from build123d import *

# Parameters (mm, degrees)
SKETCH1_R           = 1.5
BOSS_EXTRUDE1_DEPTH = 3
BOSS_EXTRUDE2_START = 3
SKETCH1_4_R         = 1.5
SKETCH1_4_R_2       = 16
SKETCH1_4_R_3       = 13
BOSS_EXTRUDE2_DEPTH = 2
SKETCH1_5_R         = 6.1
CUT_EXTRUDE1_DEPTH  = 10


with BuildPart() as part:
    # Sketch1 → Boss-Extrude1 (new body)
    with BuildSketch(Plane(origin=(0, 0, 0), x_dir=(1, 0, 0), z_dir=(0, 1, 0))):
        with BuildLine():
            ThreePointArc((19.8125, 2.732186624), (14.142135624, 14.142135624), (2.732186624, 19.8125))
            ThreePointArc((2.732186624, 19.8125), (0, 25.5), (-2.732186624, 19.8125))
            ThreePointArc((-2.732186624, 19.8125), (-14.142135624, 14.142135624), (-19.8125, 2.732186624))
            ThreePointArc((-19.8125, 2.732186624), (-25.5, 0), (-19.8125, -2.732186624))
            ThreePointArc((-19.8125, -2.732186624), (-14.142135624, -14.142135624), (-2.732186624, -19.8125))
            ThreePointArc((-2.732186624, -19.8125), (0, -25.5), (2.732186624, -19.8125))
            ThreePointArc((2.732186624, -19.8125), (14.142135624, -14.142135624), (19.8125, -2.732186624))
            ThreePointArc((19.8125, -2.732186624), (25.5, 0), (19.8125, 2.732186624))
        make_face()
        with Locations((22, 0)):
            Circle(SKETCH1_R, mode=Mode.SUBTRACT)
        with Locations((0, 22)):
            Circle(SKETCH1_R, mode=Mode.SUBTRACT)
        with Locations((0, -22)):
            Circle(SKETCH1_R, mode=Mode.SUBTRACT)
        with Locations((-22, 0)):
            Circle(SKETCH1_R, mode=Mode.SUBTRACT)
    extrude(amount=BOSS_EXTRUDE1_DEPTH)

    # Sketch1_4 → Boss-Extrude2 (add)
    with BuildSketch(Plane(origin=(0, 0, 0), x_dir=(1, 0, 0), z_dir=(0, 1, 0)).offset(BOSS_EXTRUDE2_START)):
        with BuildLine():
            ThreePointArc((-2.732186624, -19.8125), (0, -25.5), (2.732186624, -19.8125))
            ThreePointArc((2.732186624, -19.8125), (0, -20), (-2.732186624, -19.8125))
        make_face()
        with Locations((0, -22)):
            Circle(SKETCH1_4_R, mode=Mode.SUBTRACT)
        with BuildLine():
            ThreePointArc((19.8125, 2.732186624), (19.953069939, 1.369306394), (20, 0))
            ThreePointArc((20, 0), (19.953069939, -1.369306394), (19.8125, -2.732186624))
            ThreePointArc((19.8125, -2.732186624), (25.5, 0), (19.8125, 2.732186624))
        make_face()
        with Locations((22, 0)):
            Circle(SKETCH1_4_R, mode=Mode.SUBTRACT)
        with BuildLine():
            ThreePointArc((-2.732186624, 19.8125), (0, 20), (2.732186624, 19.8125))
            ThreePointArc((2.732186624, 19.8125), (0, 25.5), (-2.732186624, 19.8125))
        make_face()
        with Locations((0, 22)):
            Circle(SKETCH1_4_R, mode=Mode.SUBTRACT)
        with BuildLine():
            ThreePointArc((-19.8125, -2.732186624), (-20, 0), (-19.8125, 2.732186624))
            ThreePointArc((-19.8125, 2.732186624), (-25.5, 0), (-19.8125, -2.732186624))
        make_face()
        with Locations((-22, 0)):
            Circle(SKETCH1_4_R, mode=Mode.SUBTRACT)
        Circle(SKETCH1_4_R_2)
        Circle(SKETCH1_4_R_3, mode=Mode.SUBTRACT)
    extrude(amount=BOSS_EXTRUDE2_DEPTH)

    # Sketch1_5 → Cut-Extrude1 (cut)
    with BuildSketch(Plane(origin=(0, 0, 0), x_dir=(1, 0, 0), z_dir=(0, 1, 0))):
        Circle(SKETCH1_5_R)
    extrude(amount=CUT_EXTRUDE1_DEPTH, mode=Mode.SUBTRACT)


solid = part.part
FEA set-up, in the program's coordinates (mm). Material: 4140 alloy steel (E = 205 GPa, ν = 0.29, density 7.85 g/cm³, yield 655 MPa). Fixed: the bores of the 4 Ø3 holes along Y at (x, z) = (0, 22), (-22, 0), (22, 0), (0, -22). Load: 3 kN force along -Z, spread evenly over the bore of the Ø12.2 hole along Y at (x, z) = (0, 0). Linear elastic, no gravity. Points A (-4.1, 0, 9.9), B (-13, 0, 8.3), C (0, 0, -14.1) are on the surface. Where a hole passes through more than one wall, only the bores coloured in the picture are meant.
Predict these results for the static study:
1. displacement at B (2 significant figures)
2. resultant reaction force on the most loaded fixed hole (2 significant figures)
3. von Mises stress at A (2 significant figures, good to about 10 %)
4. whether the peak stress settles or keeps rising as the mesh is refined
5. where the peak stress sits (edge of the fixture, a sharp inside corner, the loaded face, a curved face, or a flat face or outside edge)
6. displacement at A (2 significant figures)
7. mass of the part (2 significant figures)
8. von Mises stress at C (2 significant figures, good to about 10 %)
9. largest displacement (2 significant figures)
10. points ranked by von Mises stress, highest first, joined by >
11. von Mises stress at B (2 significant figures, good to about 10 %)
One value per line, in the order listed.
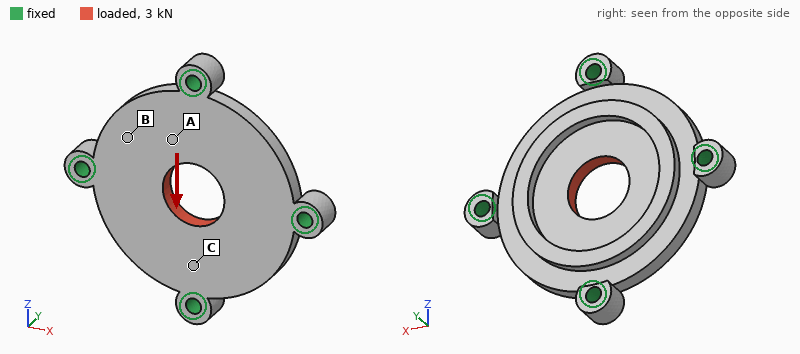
2.1 µm
1.1 kN
30 MPa
keeps rising
edge of the fixture
2.4 µm
35 g
44 MPa
3.4 µm
C > A > B
9.2 MPa
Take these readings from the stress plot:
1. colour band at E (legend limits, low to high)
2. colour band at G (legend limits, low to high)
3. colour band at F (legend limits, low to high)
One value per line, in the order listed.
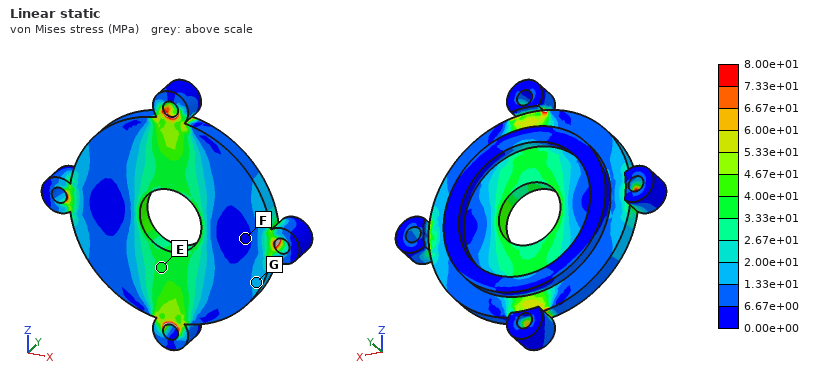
3.33e+01 to 4.00e+01 MPa
1.33e+01 to 2.00e+01 MPa
0.00e+00 to 6.67e+00 MPa
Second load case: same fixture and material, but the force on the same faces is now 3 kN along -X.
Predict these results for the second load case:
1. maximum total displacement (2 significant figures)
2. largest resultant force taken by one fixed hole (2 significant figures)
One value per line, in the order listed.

3.4 µm
1.1 kN
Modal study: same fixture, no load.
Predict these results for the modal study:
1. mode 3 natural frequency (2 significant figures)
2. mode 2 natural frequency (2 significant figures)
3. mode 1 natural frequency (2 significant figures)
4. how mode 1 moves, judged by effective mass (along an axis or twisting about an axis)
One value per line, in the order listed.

17 kHz
17 kHz
13 kHz
along Y
